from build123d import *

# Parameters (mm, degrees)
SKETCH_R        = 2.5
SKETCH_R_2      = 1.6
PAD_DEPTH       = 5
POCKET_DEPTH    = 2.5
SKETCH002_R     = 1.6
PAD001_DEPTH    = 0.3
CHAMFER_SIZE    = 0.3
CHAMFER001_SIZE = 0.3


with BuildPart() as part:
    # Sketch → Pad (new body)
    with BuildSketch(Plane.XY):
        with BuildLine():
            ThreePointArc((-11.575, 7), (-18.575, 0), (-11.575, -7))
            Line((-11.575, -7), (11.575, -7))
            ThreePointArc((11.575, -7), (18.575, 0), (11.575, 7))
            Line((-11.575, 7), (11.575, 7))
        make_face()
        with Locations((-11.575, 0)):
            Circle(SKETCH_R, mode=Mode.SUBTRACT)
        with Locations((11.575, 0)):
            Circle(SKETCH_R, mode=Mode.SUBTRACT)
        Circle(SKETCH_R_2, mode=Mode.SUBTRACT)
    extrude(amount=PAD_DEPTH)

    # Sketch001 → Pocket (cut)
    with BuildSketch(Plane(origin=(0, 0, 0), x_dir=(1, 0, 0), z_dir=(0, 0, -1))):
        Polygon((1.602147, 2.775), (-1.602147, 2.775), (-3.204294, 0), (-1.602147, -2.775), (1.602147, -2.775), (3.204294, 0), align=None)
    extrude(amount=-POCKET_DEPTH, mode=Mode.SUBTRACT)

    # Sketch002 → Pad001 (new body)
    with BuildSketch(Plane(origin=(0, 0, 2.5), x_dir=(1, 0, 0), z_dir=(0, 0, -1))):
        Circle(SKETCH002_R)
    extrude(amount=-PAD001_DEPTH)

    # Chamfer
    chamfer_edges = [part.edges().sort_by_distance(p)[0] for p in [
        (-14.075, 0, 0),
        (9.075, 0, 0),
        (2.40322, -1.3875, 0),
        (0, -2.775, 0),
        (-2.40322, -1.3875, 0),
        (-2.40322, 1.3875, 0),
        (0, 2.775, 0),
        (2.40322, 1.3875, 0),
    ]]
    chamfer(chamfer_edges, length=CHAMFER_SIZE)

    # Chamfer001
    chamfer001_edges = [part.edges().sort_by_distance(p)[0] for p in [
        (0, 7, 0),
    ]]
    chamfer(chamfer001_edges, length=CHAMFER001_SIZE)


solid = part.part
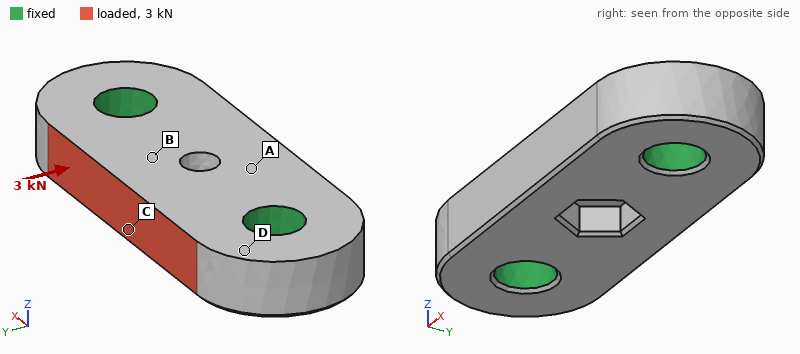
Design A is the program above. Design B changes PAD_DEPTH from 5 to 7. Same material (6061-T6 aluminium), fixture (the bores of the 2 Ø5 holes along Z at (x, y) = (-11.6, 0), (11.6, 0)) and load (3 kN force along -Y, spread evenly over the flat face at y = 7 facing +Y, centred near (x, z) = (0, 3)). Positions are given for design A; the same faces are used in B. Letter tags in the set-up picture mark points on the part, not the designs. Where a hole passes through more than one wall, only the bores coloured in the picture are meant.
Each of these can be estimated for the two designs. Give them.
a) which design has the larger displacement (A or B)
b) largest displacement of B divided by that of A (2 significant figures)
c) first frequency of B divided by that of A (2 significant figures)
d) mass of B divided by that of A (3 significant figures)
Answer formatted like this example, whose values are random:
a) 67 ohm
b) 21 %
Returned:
a) A
b) 0.71
c) 1.2
d) 1.41
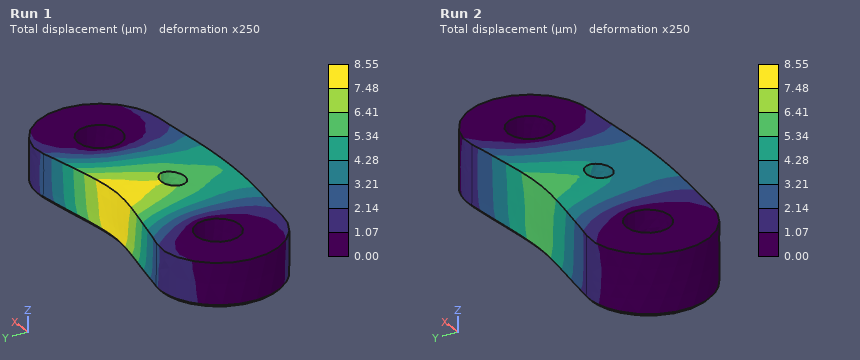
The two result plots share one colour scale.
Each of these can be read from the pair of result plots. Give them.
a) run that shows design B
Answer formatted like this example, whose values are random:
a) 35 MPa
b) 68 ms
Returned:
a) Run 2
